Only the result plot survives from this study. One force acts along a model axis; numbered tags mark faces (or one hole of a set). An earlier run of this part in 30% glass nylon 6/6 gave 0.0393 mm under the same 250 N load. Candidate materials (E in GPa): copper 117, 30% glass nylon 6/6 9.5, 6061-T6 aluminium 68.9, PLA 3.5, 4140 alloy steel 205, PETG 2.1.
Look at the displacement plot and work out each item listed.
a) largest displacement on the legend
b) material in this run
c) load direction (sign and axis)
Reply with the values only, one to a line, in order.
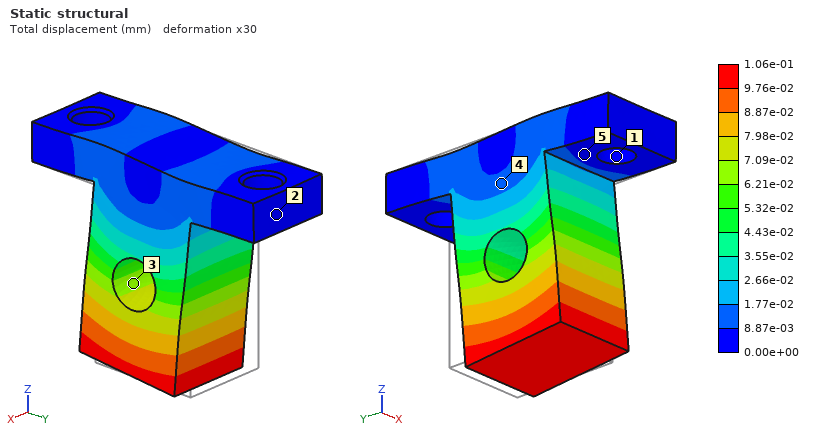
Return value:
1.06e-01 mm
PLA
-Y
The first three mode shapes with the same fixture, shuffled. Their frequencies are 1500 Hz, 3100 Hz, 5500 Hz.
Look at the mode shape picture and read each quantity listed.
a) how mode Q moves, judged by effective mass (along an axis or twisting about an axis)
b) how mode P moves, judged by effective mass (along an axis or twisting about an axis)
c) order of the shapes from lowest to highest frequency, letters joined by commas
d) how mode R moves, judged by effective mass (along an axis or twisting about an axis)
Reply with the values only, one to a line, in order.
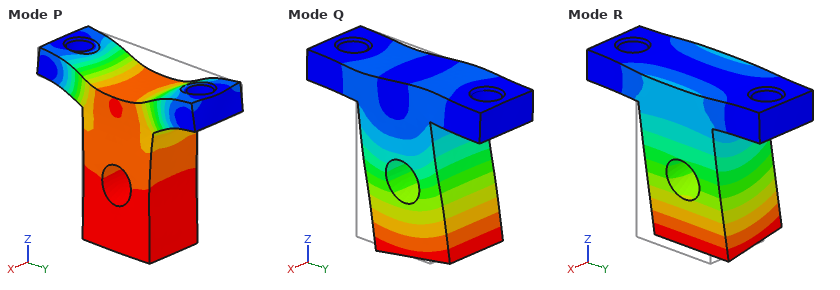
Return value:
along Y
along Z
R, Q, P
along X
